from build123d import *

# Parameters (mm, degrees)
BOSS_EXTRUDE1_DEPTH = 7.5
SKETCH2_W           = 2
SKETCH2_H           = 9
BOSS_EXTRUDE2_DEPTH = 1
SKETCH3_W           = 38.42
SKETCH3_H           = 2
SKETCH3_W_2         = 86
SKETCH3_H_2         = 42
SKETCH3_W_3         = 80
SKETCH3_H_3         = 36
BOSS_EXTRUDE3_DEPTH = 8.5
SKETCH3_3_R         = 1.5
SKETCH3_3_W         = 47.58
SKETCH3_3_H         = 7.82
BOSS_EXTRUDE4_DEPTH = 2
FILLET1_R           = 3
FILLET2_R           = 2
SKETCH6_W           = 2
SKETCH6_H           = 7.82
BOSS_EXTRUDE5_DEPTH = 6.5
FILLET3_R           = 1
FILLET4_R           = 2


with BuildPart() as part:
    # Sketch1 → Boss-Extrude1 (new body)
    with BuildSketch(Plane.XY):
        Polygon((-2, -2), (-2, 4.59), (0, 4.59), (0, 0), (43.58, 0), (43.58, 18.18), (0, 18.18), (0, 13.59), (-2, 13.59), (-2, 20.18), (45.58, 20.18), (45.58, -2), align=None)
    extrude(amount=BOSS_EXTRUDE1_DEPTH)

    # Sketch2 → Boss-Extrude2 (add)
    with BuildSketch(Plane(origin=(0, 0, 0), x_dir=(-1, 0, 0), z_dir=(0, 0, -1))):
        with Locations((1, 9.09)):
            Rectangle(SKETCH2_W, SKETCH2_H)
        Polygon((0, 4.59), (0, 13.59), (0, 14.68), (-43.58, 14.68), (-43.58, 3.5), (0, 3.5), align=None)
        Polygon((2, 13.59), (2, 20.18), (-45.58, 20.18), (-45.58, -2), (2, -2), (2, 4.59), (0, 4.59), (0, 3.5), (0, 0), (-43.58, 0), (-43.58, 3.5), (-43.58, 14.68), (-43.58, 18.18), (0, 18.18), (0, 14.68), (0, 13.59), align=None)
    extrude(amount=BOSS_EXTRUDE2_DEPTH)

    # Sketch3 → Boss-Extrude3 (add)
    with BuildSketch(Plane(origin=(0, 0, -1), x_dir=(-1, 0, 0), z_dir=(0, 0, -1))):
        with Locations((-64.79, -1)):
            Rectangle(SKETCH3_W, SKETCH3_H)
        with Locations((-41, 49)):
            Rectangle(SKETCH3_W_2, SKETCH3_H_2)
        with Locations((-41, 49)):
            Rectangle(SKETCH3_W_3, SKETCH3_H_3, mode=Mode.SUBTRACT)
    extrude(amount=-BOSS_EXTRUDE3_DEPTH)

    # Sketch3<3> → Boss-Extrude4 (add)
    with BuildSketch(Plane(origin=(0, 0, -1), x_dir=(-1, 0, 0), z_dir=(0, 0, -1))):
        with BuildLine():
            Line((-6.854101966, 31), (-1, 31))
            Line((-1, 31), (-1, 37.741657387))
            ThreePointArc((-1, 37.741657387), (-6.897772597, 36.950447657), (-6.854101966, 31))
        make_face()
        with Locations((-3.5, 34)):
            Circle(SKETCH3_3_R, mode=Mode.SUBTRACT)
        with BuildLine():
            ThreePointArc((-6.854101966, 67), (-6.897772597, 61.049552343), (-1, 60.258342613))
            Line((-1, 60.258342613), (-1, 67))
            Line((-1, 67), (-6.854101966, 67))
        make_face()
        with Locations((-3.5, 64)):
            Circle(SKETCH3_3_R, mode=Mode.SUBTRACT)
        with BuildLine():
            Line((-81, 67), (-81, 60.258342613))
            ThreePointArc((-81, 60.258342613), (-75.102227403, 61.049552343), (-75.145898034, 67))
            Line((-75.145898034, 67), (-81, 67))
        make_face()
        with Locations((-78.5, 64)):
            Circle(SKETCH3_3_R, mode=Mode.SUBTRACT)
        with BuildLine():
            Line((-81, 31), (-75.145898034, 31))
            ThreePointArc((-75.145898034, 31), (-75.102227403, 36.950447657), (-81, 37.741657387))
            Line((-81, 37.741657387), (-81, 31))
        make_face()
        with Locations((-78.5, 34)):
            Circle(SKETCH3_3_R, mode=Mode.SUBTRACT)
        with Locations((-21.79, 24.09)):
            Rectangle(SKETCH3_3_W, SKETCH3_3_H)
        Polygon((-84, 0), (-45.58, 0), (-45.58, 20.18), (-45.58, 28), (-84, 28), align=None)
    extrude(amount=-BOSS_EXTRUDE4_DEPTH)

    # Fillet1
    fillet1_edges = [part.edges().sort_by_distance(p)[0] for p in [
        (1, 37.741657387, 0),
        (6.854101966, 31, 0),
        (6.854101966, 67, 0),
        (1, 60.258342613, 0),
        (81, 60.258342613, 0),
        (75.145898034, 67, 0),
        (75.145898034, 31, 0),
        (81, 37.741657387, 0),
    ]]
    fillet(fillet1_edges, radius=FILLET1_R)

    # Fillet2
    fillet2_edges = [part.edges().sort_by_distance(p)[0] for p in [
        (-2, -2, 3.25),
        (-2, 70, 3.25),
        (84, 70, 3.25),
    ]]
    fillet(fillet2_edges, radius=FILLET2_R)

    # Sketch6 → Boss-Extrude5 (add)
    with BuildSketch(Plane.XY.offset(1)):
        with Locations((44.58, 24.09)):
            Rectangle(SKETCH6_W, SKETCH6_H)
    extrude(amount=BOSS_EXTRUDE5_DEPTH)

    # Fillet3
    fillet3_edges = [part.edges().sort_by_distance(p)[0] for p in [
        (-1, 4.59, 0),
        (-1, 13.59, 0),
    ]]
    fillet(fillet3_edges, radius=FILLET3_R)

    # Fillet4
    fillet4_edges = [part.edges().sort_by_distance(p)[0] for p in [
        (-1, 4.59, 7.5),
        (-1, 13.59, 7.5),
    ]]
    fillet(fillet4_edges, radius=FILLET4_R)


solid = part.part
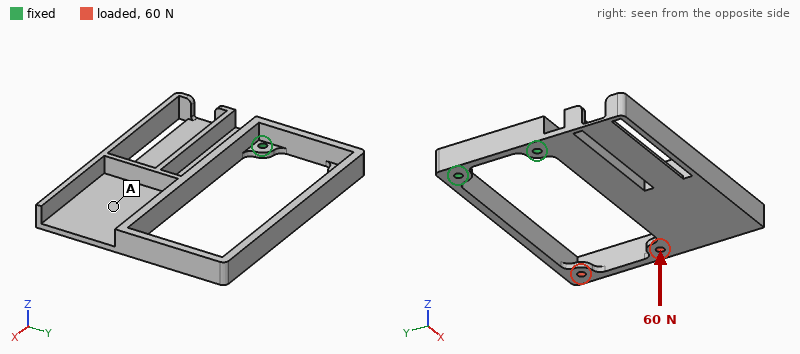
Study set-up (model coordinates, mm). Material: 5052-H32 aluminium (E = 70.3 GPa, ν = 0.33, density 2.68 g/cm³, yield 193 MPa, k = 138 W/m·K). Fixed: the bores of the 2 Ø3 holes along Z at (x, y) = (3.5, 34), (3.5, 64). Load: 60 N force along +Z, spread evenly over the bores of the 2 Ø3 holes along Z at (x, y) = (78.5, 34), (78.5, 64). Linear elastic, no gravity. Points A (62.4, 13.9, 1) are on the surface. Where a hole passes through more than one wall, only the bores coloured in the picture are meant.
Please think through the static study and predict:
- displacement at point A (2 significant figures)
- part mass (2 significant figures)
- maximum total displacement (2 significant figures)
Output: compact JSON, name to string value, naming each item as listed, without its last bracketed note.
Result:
{"displacement at point A": "0.48 mm", "part mass": "34 g", "maximum total displacement": "0.74 mm"}
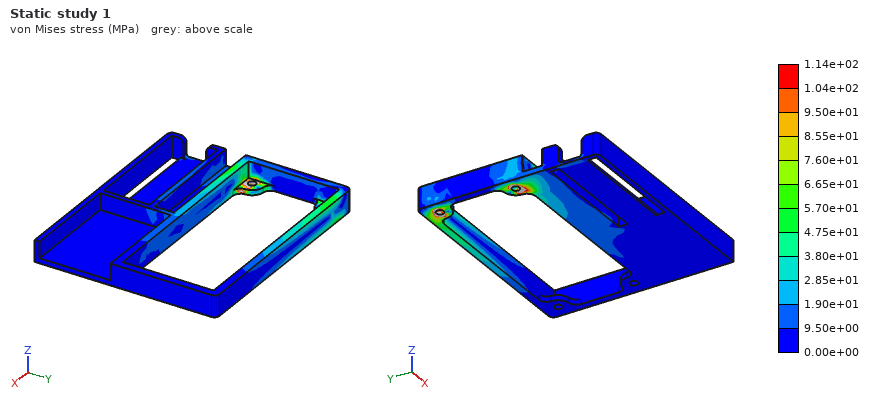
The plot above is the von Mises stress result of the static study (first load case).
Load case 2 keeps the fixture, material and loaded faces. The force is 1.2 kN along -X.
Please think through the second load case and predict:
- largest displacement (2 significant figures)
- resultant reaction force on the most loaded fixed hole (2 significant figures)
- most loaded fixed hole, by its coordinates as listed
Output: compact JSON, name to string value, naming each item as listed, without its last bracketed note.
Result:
{"largest displacement": "0.47 mm", "resultant reaction force on the most loaded fixed hole": "670 N", "most loaded fixed hole, by its coordinates as listed": "(3.5, 34)"}
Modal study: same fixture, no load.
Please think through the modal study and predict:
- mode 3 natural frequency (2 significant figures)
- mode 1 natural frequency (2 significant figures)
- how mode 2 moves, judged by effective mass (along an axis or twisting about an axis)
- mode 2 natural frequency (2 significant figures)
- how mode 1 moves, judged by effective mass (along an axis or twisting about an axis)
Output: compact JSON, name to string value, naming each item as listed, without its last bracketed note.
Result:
{"mode 3 natural frequency": "720 Hz", "mode 1 natural frequency": "360 Hz", "how mode 2 moves, judged by effective mass": "along Y", "mode 2 natural frequency": "620 Hz", "how mode 1 moves, judged by effective mass": "along Z"}
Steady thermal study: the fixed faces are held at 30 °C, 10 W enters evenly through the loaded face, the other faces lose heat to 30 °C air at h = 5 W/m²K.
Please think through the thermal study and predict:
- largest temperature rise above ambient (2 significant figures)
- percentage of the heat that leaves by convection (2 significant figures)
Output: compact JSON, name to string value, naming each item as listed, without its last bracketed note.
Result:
{"largest temperature rise above ambient": "74 K", "percentage of the heat that leaves by convection": "20 %"}
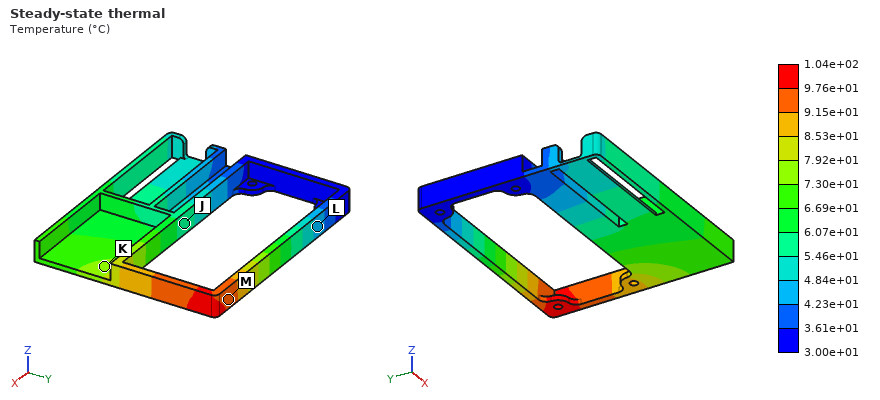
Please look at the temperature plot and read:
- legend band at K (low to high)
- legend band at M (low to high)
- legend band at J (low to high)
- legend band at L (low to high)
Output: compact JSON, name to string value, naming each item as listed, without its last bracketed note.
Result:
{"legend band at K": "7.30e+01 to 7.92e+01 °C", "legend band at M": "9.15e+01 to 9.76e+01 °C", "legend band at J": "5.46e+01 to 6.07e+01 °C", "legend band at L": "4.23e+01 to 4.84e+01 °C"}
